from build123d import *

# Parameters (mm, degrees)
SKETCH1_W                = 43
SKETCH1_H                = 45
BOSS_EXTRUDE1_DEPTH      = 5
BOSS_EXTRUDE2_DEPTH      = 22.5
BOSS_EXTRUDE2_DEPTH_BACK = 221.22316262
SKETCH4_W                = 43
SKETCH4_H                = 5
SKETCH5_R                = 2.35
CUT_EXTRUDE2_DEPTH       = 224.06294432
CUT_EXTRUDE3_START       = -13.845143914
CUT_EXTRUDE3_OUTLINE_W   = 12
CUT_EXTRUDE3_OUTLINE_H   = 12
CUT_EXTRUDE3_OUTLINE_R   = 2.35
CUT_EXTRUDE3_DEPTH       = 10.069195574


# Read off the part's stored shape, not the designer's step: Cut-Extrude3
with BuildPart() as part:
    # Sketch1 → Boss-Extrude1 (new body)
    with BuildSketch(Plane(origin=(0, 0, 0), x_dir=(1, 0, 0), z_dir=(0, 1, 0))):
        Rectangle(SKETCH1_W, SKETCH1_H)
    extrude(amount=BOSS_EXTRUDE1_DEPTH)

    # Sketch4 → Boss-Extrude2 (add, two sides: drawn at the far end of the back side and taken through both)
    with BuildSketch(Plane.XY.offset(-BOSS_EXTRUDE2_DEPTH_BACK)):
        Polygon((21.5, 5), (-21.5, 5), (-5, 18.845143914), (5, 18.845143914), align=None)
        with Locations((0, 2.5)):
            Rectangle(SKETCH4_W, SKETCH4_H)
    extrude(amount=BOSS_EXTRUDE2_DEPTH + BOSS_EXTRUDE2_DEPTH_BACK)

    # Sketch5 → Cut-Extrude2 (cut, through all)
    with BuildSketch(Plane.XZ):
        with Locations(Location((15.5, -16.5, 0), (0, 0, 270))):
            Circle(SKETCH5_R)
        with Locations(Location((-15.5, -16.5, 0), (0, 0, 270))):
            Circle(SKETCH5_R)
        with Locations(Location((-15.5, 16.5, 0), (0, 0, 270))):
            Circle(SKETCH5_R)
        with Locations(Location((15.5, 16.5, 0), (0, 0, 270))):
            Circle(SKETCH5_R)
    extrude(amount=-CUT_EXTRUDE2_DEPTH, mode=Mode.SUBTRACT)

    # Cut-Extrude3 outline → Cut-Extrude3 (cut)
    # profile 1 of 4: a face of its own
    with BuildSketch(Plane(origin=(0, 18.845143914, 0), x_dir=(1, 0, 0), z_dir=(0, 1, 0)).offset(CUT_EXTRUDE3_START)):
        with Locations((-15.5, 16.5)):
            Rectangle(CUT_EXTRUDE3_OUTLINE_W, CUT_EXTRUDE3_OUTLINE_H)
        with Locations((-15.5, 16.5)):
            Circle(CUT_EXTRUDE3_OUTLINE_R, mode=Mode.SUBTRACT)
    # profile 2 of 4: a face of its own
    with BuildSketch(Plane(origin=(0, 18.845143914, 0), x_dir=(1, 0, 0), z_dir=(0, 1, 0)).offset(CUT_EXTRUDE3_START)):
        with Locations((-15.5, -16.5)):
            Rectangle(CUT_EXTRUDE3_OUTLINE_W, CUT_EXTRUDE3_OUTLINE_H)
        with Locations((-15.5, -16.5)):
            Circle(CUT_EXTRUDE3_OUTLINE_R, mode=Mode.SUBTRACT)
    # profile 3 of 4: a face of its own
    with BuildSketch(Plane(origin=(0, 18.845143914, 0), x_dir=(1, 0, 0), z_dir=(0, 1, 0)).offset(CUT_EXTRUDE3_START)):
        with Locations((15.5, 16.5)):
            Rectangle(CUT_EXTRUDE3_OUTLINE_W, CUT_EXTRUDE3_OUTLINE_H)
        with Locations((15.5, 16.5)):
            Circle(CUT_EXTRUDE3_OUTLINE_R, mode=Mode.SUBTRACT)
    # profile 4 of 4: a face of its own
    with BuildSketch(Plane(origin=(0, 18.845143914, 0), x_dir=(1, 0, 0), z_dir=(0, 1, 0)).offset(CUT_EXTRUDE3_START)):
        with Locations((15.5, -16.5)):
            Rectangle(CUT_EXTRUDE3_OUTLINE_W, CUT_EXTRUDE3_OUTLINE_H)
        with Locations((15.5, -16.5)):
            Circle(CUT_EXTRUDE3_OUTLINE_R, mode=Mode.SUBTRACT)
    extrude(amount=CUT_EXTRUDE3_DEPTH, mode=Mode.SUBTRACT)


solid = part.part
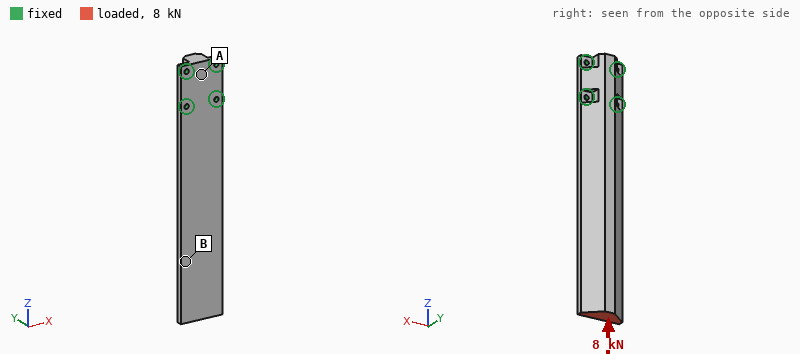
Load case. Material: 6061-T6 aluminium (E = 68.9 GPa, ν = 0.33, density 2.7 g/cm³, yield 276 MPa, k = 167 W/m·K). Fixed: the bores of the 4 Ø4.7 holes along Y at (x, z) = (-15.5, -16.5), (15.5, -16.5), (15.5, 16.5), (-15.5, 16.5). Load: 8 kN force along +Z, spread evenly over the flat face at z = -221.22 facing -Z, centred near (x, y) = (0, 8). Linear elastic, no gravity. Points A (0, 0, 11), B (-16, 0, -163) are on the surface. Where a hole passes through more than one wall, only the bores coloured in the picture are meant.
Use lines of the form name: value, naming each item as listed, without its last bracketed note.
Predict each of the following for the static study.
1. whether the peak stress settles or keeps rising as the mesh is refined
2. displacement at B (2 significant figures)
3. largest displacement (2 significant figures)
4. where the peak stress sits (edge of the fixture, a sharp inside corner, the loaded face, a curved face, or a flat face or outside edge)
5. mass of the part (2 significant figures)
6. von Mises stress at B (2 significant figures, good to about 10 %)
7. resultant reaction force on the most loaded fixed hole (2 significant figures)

whether the peak stress settles or keeps rising as the mesh is refined: keeps rising
displacement at B: 0.098 mm
largest displacement: 0.14 mm
where the peak stress sits: edge of the fixture
mass of the part: 370 g
von Mises stress at B: 14 MPa
resultant reaction force on the most loaded fixed hole: 2.9 kN
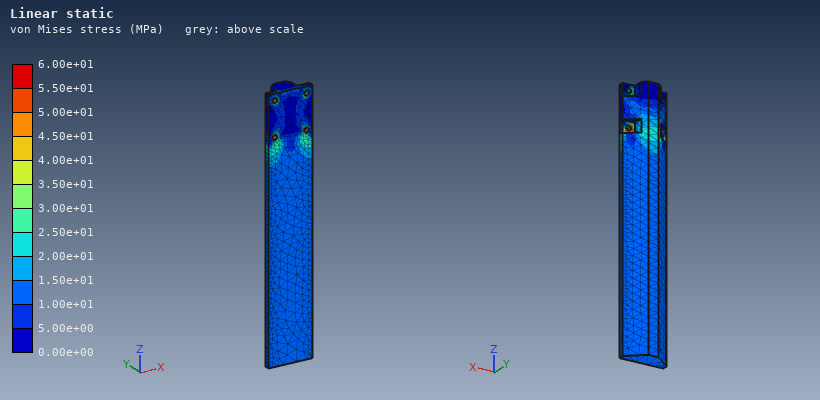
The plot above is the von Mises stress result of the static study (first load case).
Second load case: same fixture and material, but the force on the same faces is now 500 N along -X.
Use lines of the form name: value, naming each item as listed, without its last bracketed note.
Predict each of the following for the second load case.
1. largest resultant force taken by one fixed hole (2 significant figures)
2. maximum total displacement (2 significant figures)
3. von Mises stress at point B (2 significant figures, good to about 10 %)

largest resultant force taken by one fixed hole: 2.8 kN
maximum total displacement: 0.38 mm
von Mises stress at point B: 7.7 MPa
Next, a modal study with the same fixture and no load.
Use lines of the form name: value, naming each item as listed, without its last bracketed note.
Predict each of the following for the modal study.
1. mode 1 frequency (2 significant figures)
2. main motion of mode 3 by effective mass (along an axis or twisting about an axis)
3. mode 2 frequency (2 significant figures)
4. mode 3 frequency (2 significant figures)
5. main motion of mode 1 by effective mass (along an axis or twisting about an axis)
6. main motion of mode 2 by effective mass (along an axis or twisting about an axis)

mode 1 frequency: 290 Hz
main motion of mode 3 by effective mass: along Y
mode 2 frequency: 640 Hz
mode 3 frequency: 1800 Hz
main motion of mode 1 by effective mass: along Y
main motion of mode 2 by effective mass: along X
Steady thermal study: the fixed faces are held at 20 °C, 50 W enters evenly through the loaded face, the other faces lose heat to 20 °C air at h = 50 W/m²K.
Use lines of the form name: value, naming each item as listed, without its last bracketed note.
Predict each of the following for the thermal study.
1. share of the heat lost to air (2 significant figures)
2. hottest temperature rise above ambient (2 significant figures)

share of the heat lost to air: 61 %
hottest temperature rise above ambient: 64 K
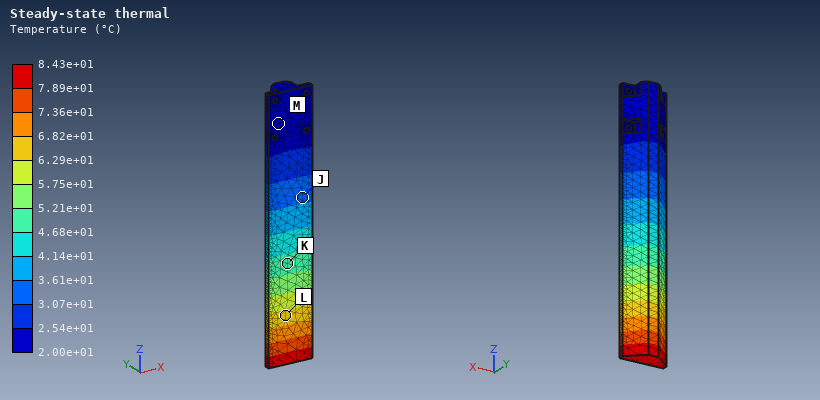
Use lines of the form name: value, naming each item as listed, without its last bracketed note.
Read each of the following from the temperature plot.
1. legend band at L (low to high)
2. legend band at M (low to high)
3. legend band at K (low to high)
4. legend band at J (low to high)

legend band at L: 6.29e+01 to 6.82e+01 °C
legend band at M: 2.00e+01 to 2.54e+01 °C
legend band at K: 4.68e+01 to 5.21e+01 °C
legend band at J: 3.07e+01 to 3.61e+01 °C
